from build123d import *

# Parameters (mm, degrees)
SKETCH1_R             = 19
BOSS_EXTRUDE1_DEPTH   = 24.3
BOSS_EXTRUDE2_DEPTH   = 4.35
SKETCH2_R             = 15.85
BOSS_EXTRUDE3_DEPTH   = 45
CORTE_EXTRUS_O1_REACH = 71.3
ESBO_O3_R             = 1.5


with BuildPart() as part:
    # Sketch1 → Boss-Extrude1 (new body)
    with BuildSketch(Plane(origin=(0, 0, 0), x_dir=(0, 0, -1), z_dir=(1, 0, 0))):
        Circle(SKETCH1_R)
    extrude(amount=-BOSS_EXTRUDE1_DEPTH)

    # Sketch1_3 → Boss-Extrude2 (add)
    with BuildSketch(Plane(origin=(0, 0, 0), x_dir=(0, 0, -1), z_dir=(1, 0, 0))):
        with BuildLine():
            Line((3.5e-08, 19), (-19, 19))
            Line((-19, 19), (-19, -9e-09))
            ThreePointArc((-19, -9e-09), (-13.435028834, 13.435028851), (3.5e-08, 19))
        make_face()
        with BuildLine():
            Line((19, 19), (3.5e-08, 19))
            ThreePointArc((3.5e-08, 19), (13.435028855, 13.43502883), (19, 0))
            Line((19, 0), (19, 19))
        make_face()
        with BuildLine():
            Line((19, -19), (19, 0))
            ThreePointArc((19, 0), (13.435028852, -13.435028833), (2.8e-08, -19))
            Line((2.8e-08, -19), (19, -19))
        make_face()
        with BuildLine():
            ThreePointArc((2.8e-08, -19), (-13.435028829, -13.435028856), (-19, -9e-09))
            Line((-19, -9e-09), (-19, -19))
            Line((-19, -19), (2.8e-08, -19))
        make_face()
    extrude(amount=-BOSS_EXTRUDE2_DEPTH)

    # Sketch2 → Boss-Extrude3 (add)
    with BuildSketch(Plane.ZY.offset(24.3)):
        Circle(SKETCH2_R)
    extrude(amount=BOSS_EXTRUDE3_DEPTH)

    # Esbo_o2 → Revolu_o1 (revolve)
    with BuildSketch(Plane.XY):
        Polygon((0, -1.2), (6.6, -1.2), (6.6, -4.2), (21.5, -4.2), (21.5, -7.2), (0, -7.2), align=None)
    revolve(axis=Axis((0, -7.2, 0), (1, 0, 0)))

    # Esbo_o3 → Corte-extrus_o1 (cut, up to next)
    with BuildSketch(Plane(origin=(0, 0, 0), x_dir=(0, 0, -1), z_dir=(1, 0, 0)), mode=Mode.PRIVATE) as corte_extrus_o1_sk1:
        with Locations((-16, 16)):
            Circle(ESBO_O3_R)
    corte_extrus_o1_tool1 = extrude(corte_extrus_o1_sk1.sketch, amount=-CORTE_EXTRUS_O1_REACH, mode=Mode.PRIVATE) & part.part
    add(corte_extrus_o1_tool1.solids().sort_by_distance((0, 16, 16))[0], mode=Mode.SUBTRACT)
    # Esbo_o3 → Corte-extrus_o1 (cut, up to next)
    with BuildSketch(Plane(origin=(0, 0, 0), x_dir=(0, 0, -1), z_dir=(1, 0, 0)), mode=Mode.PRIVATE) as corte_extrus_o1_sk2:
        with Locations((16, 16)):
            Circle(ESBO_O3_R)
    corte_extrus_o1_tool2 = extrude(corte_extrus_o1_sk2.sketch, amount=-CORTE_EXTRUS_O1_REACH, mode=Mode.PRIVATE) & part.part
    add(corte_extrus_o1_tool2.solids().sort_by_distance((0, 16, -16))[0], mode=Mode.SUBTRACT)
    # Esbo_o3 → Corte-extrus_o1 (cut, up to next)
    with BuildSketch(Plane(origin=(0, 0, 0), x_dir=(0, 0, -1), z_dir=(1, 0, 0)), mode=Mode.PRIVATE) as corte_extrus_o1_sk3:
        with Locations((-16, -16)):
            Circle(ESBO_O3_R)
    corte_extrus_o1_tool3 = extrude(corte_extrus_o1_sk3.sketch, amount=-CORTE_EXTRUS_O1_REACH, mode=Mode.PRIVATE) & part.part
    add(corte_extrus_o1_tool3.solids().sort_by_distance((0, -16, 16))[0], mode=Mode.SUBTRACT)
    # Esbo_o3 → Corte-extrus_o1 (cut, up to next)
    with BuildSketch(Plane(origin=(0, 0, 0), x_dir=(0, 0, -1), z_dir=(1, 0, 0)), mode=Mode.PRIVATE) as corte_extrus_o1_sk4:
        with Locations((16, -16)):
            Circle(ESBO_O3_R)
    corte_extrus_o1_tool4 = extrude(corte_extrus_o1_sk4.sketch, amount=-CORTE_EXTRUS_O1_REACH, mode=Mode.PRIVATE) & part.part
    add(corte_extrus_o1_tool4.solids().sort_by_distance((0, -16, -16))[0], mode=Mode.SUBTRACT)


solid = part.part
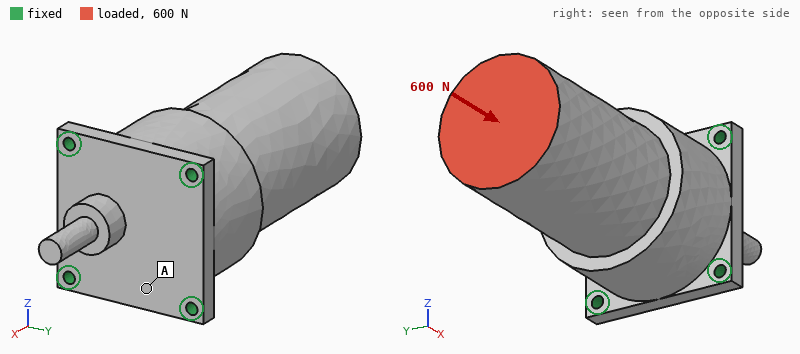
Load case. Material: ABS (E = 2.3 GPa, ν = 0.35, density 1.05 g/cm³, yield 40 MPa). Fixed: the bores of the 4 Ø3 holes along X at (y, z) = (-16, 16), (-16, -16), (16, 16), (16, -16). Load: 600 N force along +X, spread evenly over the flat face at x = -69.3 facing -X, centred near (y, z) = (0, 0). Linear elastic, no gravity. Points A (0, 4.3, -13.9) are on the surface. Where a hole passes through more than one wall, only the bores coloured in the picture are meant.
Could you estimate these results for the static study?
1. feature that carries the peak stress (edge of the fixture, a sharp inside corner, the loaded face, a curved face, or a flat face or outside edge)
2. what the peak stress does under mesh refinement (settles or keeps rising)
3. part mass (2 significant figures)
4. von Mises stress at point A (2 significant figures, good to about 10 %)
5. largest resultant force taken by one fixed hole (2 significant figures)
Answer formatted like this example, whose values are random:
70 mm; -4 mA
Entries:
edge of the fixture; keeps rising; 69 g; 1.5 MPa; 160 N
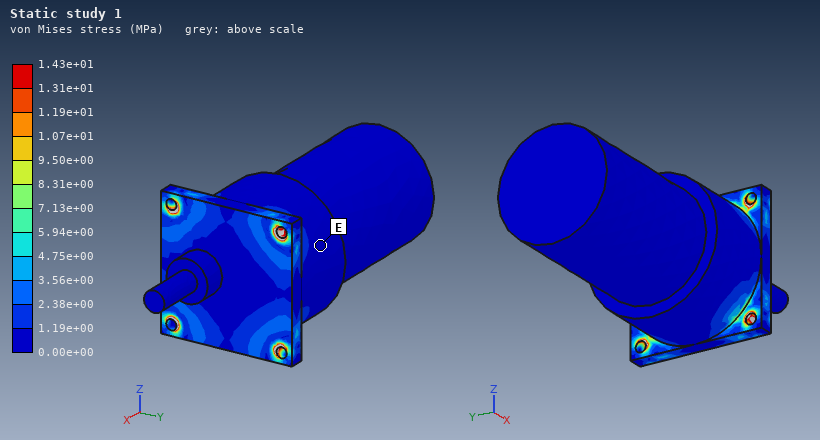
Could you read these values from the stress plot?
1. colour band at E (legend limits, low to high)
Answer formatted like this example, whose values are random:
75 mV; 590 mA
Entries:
0.00e+00 to 1.19e+00 MPa
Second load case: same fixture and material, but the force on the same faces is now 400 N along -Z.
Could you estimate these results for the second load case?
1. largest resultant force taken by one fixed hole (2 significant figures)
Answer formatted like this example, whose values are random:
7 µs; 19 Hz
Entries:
490 N
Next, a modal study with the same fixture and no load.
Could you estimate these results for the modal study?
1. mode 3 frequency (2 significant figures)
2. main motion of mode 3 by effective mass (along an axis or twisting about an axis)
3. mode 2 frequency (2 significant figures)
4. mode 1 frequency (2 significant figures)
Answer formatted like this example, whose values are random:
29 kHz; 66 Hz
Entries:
2300 Hz; along X; 850 Hz; 850 Hz
